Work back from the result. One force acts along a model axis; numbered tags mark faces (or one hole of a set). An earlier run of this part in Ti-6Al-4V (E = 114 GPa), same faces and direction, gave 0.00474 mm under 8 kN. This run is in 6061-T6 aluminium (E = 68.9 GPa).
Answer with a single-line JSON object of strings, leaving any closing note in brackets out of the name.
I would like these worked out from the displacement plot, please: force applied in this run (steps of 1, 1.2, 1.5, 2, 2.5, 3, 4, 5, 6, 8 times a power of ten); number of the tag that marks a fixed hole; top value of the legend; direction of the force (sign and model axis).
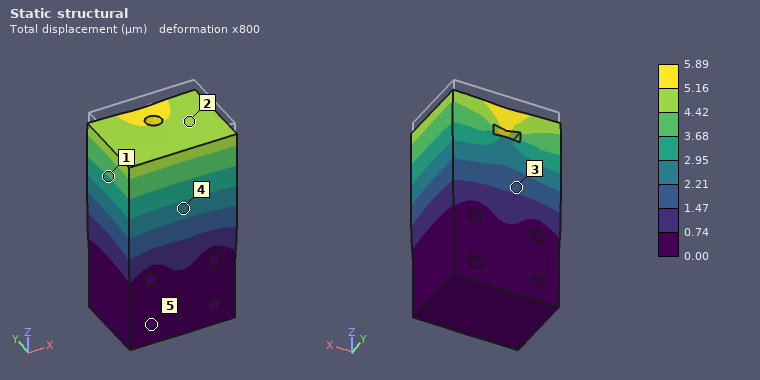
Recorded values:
{"force applied in this run": "6 kN", "number of the tag that marks a fixed hole": "5", "top value of the legend": "5.89 µm", "direction of the force": "-Z"}
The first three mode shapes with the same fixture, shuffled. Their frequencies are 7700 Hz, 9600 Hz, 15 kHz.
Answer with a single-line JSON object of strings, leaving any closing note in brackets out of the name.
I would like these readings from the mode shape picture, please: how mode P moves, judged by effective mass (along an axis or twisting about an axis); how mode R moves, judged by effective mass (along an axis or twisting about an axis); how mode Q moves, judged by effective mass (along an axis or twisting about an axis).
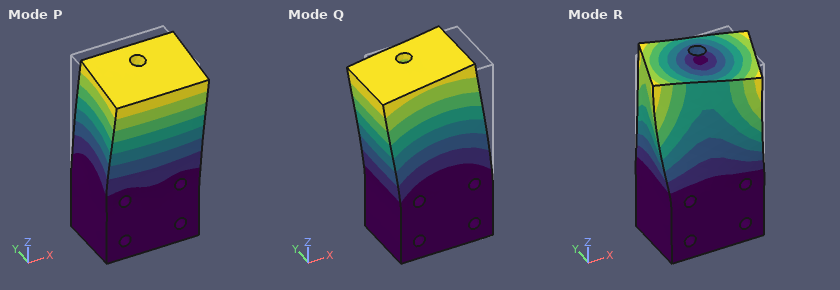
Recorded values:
{"how mode P moves, judged by effective mass": "along Y", "how mode R moves, judged by effective mass": "twisting about Z", "how mode Q moves, judged by effective mass": "along X"}
